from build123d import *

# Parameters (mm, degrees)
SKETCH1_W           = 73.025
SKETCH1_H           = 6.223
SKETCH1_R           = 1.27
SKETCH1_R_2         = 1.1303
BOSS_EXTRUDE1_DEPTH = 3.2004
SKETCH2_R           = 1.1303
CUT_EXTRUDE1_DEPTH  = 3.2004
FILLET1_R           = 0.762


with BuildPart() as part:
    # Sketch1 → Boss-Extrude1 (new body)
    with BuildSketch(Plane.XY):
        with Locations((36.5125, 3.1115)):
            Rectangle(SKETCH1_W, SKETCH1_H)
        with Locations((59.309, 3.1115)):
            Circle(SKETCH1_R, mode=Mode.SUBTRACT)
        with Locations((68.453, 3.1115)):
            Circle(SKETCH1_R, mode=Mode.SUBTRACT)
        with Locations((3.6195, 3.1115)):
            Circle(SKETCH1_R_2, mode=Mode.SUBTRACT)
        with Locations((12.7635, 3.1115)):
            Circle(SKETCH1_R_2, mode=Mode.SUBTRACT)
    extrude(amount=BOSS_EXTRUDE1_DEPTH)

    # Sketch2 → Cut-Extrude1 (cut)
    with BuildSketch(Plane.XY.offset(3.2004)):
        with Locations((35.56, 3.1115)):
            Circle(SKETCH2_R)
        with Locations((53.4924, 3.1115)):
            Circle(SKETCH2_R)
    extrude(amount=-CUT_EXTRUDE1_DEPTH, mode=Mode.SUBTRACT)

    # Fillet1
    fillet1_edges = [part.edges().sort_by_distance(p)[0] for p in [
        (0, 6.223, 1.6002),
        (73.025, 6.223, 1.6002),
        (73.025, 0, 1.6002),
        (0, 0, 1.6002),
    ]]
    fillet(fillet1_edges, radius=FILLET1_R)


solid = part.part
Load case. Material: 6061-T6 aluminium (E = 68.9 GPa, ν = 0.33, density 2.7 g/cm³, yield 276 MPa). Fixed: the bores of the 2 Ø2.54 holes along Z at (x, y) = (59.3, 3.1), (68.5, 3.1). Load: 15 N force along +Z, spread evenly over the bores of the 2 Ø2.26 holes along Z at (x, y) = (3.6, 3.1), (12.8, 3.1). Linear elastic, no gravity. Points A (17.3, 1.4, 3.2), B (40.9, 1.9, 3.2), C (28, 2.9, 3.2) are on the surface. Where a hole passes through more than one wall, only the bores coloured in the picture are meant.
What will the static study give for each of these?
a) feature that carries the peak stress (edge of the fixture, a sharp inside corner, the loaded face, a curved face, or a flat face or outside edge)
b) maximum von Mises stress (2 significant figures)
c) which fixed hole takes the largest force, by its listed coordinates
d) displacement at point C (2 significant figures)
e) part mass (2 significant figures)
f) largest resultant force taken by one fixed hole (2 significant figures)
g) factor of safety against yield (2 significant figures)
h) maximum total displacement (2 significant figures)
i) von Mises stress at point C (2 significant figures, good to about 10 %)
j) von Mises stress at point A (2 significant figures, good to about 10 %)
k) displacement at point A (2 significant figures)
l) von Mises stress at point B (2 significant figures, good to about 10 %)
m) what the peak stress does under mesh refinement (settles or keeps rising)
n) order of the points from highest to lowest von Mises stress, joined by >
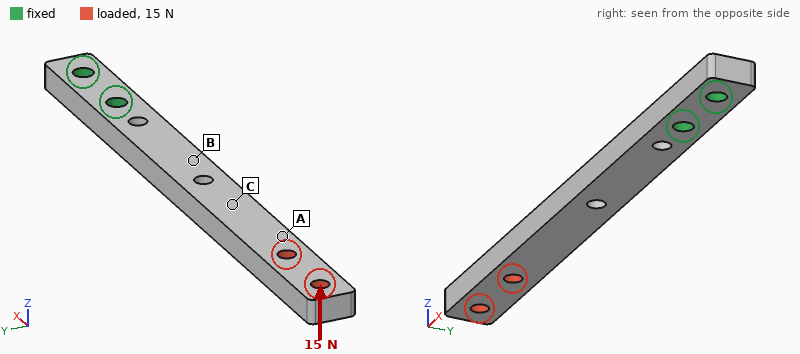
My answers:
a curved face
160 MPa
(59.3, 3.1)
0.28 mm
3.7 g
22 N
1.7
0.77 mm
28 MPa
13 MPa
0.45 mm
46 MPa
settles
B > C > A
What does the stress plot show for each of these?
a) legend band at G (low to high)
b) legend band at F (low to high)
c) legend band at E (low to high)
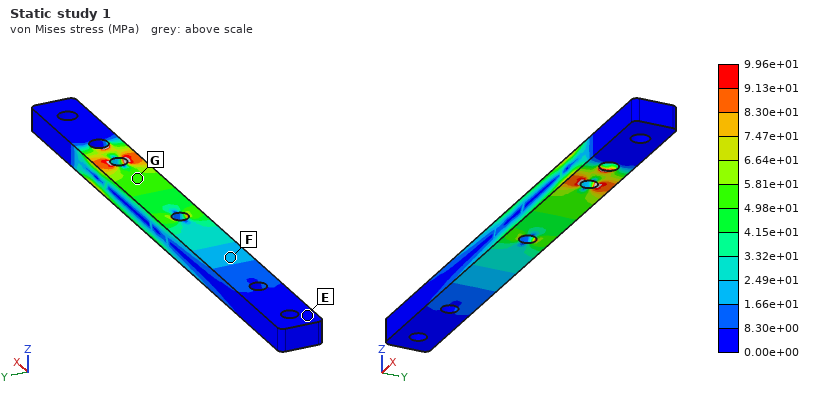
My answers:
4.98e+01 to 5.81e+01 MPa
1.66e+01 to 2.49e+01 MPa
0.00e+00 to 8.30e+00 MPa
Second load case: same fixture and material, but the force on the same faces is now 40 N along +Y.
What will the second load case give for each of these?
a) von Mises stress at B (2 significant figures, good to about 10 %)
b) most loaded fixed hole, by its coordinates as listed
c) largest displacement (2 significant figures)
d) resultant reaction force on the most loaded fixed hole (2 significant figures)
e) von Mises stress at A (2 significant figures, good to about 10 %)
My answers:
25 MPa
(59.3, 3.1)
0.54 mm
110 N
10 MPa
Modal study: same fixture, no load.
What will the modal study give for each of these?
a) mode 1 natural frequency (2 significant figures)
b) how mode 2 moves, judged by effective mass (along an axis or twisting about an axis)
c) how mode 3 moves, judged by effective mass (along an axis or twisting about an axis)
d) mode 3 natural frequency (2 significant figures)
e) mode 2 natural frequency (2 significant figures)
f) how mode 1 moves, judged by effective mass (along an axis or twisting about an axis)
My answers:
740 Hz
along Y
along Z
4600 Hz
1400 Hz
along Z
